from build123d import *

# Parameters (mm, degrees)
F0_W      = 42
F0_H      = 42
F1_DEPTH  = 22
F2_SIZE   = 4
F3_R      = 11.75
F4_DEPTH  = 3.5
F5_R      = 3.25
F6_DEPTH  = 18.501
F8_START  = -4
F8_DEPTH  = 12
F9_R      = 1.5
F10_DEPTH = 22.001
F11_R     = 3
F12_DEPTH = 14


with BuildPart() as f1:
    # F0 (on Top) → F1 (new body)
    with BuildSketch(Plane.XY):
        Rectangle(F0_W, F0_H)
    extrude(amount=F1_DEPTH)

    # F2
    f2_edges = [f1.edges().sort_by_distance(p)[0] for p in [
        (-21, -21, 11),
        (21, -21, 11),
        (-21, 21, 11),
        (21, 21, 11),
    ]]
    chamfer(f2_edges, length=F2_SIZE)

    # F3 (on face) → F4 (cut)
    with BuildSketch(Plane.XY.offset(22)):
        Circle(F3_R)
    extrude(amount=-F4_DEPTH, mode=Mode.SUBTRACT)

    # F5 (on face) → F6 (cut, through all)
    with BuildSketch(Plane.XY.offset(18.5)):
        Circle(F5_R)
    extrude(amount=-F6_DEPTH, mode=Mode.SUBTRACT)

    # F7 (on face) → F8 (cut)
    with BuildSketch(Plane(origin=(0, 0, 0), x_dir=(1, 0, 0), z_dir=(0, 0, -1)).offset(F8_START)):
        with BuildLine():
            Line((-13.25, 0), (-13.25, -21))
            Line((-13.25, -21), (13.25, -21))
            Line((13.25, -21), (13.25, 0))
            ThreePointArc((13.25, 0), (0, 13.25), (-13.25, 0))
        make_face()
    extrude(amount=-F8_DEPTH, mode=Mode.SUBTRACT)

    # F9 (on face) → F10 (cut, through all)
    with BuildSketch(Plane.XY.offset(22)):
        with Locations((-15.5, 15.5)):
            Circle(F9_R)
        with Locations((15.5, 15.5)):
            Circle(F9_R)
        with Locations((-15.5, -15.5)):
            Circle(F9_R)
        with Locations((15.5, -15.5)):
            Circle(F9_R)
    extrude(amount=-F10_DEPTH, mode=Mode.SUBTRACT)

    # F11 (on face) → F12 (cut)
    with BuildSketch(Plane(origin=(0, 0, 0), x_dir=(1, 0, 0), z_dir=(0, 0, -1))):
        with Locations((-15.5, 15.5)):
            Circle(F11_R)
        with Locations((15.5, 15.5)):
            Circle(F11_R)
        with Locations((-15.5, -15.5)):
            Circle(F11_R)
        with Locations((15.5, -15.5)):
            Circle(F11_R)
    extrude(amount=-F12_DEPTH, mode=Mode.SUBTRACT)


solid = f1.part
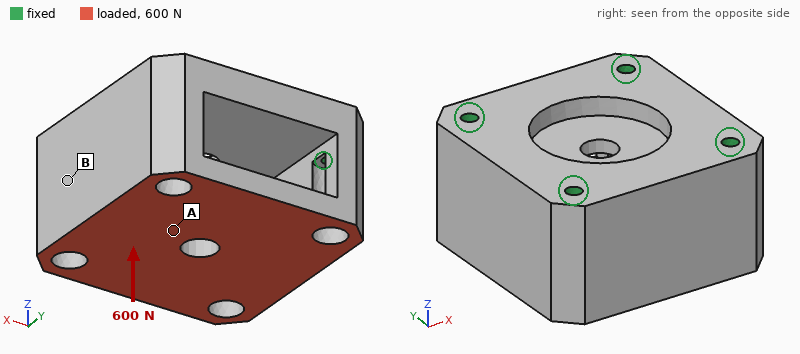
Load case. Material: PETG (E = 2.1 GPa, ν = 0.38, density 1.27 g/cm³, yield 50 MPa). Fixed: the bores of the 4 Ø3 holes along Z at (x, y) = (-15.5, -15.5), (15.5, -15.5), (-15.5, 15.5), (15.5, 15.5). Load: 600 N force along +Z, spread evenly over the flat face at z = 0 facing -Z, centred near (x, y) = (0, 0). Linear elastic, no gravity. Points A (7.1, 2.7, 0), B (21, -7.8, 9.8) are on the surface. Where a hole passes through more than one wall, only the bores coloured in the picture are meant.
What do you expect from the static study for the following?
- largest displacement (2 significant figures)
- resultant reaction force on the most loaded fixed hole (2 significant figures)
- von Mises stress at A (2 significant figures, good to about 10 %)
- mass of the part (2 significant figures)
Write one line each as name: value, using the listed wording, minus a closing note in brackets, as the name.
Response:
largest displacement: 0.16 mm
resultant reaction force on the most loaded fixed hole: 160 N
von Mises stress at A: 1.5 MPa
mass of the part: 31 g
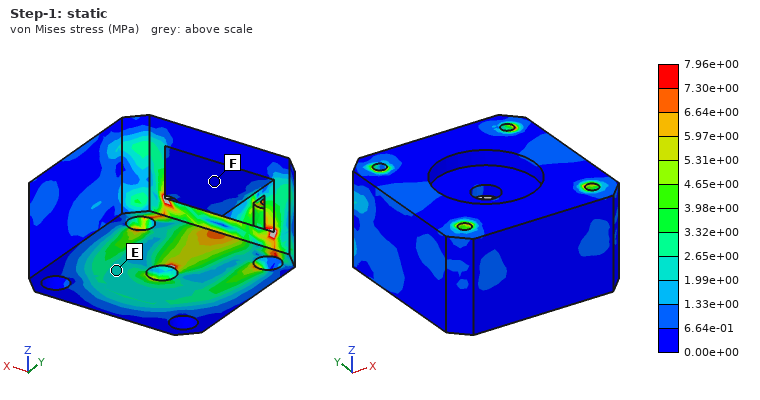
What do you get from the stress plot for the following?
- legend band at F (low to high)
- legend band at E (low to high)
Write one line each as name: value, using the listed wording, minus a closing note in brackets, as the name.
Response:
legend band at F: 0.00e+00 to 6.64e-01 MPa
legend band at E: 1.99e+00 to 2.65e+00 MPa
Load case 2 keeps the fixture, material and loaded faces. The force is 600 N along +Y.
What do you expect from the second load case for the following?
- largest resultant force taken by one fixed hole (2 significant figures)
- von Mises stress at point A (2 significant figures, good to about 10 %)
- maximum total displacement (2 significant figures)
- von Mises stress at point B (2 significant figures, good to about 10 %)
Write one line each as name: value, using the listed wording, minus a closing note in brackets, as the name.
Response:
largest resultant force taken by one fixed hole: 220 N
von Mises stress at point A: 1.5 MPa
maximum total displacement: 85 µm
von Mises stress at point B: 1.9 MPa
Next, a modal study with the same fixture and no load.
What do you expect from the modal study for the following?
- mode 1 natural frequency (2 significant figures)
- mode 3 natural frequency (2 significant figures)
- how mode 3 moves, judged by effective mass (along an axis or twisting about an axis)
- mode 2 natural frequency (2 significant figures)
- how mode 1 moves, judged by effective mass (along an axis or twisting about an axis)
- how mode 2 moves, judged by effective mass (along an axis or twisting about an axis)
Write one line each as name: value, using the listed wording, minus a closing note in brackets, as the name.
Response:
mode 1 natural frequency: 3900 Hz
mode 3 natural frequency: 5500 Hz
how mode 3 moves, judged by effective mass: along Y
mode 2 natural frequency: 4400 Hz
how mode 1 moves, judged by effective mass: along X
how mode 2 moves, judged by effective mass: along Z
